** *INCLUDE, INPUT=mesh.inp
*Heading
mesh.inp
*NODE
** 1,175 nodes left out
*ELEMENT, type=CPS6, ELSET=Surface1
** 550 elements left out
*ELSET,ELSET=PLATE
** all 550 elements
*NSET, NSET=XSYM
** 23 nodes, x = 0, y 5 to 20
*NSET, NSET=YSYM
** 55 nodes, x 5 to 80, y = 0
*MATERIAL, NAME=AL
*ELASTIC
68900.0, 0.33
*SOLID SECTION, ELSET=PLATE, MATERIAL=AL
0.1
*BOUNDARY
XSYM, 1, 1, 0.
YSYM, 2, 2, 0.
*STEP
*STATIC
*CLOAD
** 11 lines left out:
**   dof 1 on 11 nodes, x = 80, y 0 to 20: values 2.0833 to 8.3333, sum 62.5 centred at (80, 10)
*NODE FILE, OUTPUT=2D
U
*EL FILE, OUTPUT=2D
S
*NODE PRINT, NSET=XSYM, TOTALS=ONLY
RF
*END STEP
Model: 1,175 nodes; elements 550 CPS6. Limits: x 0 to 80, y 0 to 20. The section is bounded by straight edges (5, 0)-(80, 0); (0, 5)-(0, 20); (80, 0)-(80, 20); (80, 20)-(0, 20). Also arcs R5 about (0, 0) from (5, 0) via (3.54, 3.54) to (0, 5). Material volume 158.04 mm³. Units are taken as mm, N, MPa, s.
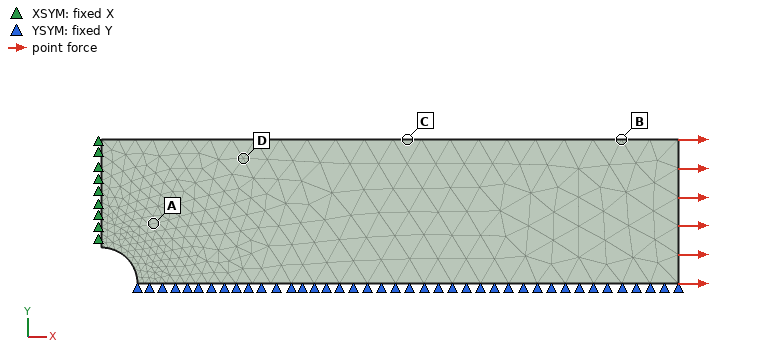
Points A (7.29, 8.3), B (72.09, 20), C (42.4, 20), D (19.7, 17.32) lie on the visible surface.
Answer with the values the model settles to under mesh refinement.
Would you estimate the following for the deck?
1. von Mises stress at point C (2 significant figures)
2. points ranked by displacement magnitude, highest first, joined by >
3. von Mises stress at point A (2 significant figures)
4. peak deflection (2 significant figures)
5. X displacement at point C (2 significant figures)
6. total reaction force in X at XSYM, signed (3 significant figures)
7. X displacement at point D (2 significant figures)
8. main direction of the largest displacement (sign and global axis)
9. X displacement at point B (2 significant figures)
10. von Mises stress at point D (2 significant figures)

31 MPa
B > C > D > A
42 MPa
0.039 mm
0.021 mm
-62.5 N
0.0099 mm
+X
0.034 mm
35 MPa
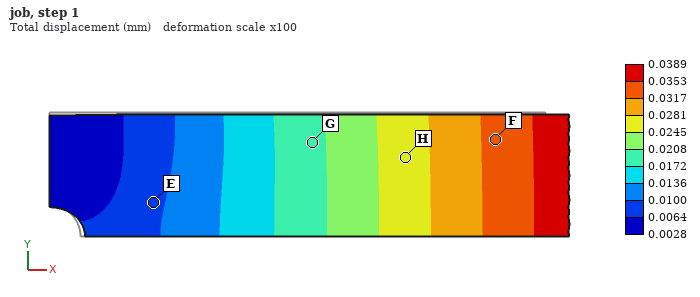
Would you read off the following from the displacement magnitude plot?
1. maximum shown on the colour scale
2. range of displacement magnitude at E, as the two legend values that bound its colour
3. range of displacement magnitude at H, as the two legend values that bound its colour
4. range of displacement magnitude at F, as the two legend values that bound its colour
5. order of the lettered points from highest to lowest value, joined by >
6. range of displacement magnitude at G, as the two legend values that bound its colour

0.0389 mm
0.0064 to 0.0100 mm
0.0245 to 0.0281 mm
0.0317 to 0.0353 mm
F > H > G > E
0.0172 to 0.0208 mm
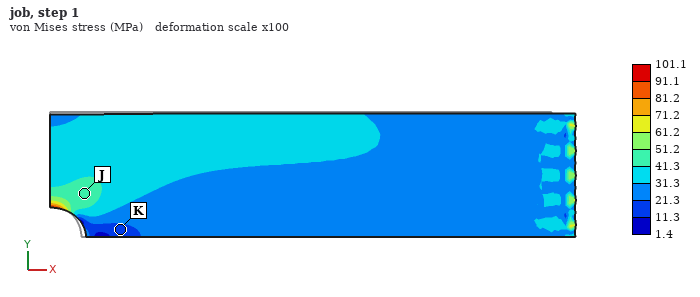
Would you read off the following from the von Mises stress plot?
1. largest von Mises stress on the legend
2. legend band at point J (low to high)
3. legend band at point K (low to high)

101.1 MPa
41.3 to 51.2 MPa
11.3 to 21.3 MPa
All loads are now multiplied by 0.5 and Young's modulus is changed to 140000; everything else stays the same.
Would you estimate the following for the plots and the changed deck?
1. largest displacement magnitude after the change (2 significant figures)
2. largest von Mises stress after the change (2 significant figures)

0.0096 mm
51 MPa
